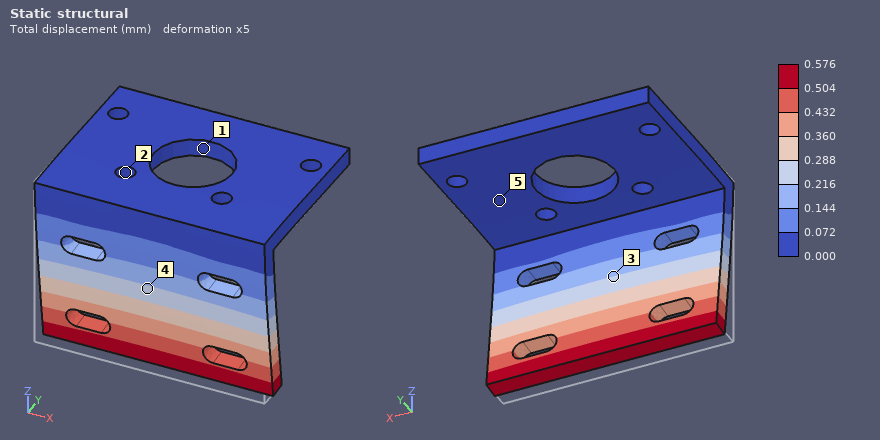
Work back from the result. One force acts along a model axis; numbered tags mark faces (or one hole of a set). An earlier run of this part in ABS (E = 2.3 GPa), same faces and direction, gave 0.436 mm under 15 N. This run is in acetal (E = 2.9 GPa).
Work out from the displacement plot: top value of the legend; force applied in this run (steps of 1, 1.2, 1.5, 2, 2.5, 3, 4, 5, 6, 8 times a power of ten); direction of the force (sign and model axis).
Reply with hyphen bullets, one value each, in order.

- 0.576 mm
- 25 N
- +Y
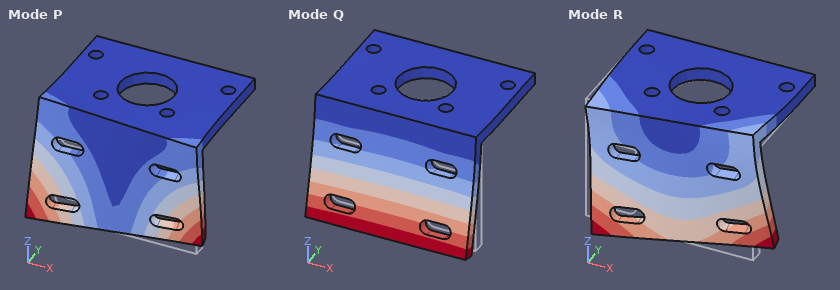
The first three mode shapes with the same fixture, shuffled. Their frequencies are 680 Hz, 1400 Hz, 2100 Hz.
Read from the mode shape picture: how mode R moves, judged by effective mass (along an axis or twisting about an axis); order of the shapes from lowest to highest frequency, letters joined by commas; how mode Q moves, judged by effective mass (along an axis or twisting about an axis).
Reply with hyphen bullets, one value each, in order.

- along X
- Q, P, R
- along Y
